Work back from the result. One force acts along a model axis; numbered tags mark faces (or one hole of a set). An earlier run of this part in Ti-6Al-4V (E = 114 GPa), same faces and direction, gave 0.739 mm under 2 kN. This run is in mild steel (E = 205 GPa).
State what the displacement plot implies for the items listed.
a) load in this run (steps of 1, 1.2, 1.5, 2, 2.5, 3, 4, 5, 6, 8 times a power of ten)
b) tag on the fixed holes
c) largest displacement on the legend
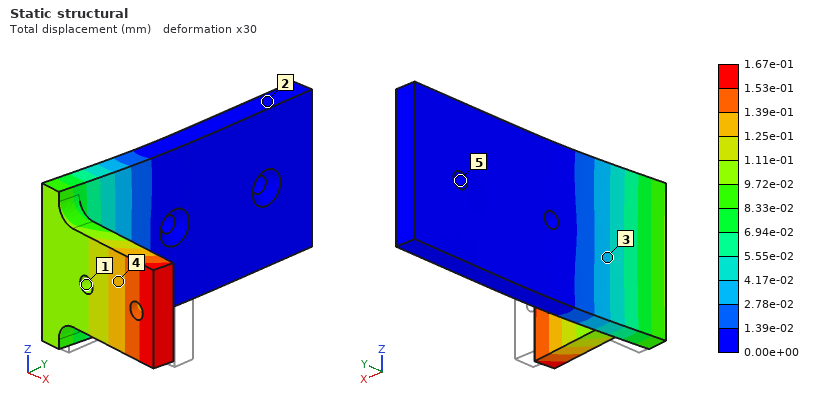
800 N
5
1.67e-01 mm
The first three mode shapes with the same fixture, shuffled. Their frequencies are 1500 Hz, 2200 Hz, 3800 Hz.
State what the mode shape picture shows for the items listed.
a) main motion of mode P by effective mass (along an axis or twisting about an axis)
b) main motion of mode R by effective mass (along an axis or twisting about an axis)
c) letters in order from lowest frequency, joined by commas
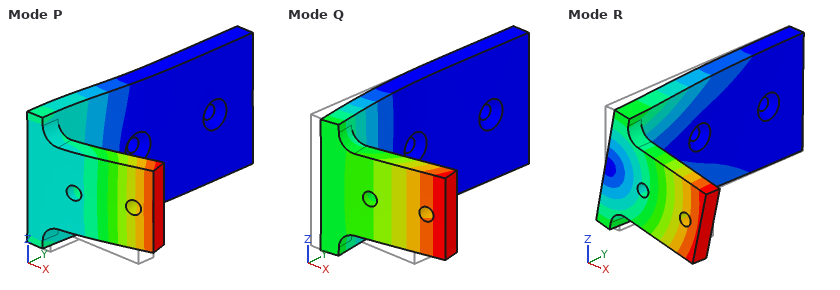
along X
along Z
Q, R, P
